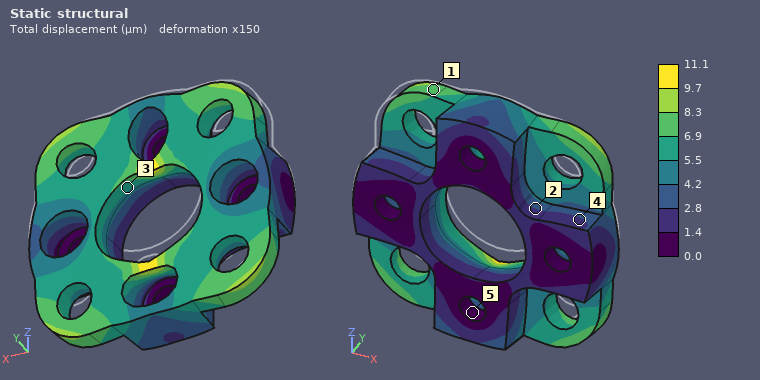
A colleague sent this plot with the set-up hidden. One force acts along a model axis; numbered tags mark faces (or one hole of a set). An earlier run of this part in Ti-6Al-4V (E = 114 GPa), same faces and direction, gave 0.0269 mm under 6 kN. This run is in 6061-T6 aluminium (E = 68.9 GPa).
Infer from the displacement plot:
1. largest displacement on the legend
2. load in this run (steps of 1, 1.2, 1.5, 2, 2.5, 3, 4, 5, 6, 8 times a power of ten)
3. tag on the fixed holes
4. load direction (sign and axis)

11.1 µm
1.5 kN
5
-Z
